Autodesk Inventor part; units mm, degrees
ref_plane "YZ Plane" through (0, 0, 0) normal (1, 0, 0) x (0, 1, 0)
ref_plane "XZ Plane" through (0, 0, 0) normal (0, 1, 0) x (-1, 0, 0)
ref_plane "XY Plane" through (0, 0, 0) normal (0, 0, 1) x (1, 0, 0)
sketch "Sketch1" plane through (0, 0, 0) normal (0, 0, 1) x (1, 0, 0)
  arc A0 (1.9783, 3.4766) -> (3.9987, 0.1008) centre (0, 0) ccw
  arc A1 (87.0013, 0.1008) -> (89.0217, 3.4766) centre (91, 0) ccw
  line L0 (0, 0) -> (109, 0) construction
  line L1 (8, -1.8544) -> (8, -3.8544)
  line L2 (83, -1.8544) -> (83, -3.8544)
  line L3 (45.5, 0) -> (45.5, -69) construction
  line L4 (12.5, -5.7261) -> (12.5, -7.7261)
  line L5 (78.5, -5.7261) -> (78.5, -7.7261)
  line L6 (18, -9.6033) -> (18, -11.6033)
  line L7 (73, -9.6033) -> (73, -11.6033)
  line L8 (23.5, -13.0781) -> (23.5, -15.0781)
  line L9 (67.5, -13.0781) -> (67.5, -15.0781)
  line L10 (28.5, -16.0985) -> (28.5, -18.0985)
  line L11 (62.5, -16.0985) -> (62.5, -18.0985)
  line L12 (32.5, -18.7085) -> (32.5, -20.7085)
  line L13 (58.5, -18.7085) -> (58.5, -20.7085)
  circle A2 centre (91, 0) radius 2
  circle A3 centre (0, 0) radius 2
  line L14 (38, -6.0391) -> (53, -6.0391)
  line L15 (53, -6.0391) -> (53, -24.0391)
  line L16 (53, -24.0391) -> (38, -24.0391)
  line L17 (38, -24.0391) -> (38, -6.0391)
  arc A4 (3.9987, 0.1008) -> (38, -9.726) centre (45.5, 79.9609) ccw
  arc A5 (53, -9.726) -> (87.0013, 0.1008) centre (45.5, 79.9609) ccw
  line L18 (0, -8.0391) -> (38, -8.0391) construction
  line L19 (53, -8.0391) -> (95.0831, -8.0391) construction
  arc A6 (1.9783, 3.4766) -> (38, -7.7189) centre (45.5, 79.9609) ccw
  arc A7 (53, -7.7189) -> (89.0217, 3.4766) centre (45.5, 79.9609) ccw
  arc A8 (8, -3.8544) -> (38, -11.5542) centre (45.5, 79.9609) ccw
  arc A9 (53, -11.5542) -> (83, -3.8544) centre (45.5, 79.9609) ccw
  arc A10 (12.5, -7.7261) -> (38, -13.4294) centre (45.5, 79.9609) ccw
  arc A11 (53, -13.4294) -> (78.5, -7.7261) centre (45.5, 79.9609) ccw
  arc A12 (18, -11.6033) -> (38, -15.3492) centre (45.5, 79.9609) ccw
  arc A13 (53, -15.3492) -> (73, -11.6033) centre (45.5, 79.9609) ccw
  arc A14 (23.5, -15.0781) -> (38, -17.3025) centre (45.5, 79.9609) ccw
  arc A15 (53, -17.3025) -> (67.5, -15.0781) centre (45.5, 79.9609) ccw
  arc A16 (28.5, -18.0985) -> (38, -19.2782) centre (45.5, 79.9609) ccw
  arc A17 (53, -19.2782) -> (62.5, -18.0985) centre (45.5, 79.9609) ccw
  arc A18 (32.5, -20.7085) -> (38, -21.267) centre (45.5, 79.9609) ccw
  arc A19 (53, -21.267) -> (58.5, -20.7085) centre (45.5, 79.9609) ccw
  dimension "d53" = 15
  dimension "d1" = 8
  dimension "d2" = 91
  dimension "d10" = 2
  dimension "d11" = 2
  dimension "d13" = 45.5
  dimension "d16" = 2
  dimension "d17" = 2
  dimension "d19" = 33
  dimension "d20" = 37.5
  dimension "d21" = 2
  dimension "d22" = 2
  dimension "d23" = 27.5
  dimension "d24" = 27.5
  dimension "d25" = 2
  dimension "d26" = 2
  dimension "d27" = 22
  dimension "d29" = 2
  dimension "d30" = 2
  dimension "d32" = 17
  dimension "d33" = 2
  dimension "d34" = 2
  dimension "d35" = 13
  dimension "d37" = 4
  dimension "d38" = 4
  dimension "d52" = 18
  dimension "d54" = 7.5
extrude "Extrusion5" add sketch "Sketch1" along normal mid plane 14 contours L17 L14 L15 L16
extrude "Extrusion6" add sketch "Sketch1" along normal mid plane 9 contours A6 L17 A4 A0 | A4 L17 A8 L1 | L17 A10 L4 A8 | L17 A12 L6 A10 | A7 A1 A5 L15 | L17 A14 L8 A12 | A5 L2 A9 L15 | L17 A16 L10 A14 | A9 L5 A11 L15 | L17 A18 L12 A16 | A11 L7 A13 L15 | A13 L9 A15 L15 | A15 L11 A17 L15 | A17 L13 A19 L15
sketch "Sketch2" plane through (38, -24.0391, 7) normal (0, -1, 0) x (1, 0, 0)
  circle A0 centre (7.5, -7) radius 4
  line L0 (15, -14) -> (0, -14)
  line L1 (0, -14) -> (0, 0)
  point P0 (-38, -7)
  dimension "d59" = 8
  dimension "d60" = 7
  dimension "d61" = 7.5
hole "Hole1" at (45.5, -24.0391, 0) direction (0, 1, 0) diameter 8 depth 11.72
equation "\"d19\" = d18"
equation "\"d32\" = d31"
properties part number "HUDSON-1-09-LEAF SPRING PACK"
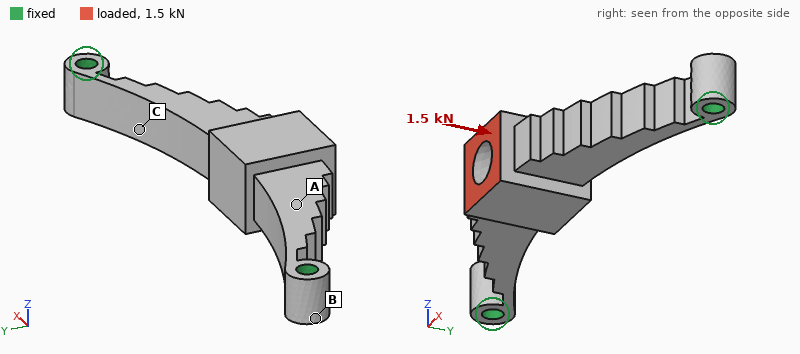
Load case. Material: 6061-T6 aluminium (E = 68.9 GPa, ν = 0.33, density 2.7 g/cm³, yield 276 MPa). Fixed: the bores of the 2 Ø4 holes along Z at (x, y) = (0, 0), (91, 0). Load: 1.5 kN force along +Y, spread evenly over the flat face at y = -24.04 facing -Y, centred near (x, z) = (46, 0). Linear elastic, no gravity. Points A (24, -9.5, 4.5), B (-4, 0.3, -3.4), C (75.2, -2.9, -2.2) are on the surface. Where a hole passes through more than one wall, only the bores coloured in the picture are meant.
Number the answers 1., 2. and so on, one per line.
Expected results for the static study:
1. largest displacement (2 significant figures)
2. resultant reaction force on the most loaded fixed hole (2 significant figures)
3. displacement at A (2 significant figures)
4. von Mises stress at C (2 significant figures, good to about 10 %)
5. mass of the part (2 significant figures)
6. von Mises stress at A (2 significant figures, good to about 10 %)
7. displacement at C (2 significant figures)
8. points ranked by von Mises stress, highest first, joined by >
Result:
1. 57 µm
2. 1.5 kN
3. 42 µm
4. 37 MPa
5. 24 g
6. 22 MPa
7. 29 µm
8. C > A > B
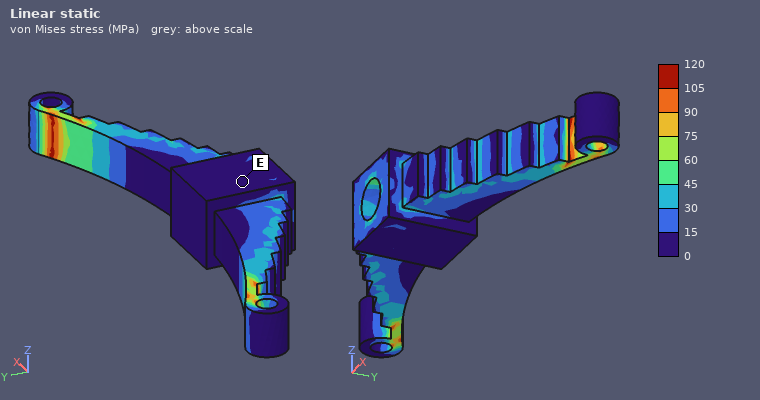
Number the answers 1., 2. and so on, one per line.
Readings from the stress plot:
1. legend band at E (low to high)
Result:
1. 0 to 15 MPa
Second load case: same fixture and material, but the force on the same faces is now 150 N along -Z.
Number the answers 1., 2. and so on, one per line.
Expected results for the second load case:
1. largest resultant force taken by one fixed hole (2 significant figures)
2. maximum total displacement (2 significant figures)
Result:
1. 75 N
2. 0.20 mm
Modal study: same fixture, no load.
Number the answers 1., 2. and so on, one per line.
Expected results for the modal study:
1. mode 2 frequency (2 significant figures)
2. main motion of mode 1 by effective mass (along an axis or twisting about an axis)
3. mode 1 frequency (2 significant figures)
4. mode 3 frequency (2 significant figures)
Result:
1. 6300 Hz
2. along Z
3. 1700 Hz
4. 6300 Hz
